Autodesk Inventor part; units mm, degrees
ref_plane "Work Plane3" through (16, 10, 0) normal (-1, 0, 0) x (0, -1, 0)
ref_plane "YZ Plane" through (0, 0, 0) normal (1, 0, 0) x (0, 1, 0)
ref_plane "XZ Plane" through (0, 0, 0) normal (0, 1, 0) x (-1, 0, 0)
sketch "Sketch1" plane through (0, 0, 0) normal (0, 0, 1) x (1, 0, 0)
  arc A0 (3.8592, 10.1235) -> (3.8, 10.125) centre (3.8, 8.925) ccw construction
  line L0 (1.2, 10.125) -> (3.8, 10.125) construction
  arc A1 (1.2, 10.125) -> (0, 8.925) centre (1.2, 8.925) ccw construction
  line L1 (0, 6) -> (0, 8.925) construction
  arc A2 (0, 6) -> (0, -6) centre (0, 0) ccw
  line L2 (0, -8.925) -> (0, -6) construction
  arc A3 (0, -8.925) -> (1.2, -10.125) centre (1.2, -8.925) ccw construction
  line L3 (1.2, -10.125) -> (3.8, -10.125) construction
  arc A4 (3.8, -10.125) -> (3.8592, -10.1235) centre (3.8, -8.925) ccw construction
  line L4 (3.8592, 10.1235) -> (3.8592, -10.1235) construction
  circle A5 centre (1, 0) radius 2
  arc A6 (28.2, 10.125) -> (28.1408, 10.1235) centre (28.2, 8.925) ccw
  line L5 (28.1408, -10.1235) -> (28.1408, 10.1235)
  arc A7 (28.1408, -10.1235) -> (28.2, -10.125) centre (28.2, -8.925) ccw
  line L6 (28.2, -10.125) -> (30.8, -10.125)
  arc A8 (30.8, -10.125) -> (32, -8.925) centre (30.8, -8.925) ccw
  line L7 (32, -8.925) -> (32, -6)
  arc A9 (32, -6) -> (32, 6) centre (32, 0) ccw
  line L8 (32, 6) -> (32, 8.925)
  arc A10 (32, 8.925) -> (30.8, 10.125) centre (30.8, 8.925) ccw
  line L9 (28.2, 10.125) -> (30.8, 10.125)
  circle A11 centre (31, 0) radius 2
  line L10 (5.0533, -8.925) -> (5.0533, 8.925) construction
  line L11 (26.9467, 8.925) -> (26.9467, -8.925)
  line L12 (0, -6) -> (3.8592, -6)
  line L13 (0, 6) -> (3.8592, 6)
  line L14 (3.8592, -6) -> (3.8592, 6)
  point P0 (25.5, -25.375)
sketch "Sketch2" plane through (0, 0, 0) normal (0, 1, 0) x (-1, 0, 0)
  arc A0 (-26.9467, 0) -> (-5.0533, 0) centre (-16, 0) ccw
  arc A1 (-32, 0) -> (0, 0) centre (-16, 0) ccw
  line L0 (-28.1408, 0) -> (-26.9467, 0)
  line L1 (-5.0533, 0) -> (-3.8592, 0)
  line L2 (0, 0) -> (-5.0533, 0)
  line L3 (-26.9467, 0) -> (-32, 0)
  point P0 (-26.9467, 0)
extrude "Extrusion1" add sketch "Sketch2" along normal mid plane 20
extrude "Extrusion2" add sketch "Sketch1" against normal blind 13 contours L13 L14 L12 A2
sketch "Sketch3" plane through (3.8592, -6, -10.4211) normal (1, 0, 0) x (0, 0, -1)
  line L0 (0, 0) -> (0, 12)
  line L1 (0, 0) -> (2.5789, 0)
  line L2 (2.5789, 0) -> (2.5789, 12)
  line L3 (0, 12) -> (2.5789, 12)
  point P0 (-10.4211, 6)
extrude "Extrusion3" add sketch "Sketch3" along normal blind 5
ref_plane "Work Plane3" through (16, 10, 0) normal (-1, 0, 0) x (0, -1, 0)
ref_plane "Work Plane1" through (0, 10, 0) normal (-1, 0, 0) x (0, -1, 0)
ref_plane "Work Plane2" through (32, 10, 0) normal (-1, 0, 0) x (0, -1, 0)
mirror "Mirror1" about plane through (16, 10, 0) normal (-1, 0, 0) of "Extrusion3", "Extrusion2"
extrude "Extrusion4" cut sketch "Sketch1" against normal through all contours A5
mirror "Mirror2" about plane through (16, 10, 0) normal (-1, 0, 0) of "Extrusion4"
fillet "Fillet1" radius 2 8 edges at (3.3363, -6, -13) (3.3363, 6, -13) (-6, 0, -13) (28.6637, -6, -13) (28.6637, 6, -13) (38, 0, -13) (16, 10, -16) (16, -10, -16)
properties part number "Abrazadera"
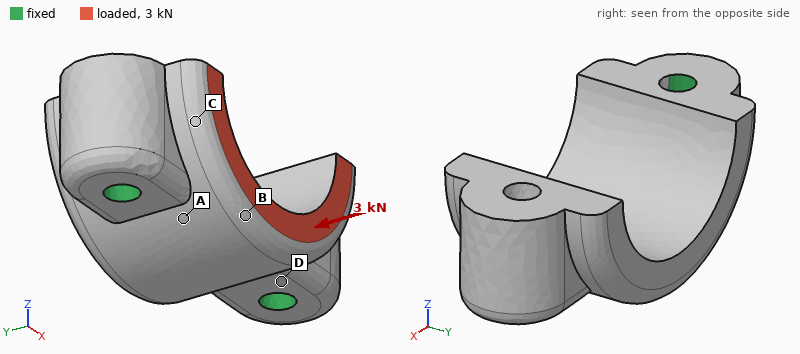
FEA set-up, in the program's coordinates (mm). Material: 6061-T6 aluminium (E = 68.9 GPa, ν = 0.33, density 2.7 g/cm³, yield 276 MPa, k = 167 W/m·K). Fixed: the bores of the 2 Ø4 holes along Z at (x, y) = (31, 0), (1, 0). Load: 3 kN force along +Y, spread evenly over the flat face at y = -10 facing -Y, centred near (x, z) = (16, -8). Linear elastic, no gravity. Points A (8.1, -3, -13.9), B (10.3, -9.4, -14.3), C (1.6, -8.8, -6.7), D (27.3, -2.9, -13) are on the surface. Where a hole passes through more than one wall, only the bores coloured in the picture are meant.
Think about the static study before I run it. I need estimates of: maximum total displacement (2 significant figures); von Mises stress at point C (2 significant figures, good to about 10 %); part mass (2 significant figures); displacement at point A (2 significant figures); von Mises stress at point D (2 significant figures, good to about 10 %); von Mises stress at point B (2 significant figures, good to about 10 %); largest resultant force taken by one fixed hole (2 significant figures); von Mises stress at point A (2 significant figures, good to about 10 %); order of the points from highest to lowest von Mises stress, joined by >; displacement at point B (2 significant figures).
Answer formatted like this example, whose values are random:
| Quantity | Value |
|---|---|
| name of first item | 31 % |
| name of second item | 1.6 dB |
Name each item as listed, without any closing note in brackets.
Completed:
| Quantity | Value |
|---|---|
| maximum total displacement | 12 µm |
| von Mises stress at point C | 7.0 MPa |
| part mass | 16 g |
| displacement at point A | 6.1 µm |
| von Mises stress at point D | 34 MPa |
| von Mises stress at point B | 13 MPa |
| largest resultant force taken by one fixed hole | 1.5 kN |
| von Mises stress at point A | 24 MPa |
| order of the points from highest to lowest von Mises stress, joined by > | D > A > B > C |
| displacement at point B | 7.7 µm |
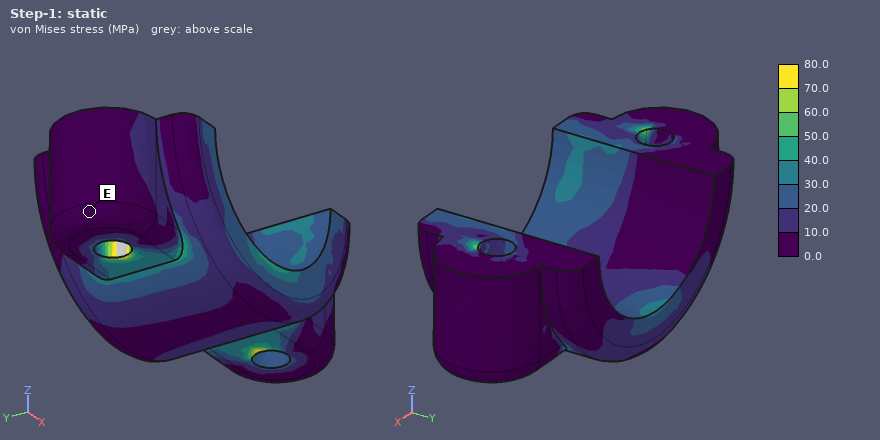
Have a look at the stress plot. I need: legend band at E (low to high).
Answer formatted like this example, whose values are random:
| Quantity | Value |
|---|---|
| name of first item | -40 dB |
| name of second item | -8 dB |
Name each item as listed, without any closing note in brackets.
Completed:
| Quantity | Value |
|---|---|
| legend band at E | 0.0 to 10.0 MPa |
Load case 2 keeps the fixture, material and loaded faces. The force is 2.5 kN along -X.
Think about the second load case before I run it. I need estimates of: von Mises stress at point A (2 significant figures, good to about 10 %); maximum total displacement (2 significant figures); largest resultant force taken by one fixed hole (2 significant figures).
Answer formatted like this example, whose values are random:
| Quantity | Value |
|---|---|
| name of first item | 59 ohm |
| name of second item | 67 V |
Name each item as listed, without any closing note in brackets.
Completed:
| Quantity | Value |
|---|---|
| von Mises stress at point A | 15 MPa |
| maximum total displacement | 15 µm |
| largest resultant force taken by one fixed hole | 1.4 kN |
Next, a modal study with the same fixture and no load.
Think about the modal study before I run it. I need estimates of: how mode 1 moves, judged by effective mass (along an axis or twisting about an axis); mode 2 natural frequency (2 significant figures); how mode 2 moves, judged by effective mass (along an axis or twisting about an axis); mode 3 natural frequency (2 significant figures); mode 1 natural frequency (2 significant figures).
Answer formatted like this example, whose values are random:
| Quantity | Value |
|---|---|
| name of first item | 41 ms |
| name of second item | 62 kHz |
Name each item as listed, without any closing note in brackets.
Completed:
| Quantity | Value |
|---|---|
| how mode 1 moves, judged by effective mass | along Y |
| mode 2 natural frequency | 36 kHz |
| how mode 2 moves, judged by effective mass | along Z |
| mode 3 natural frequency | 41 kHz |
| mode 1 natural frequency | 29 kHz |
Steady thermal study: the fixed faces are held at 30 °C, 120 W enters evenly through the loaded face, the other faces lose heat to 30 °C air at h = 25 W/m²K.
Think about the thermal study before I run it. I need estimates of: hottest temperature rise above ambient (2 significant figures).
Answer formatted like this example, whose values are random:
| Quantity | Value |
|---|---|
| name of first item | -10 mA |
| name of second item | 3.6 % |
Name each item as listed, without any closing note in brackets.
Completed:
| Quantity | Value |
|---|---|
| hottest temperature rise above ambient | 51 K |
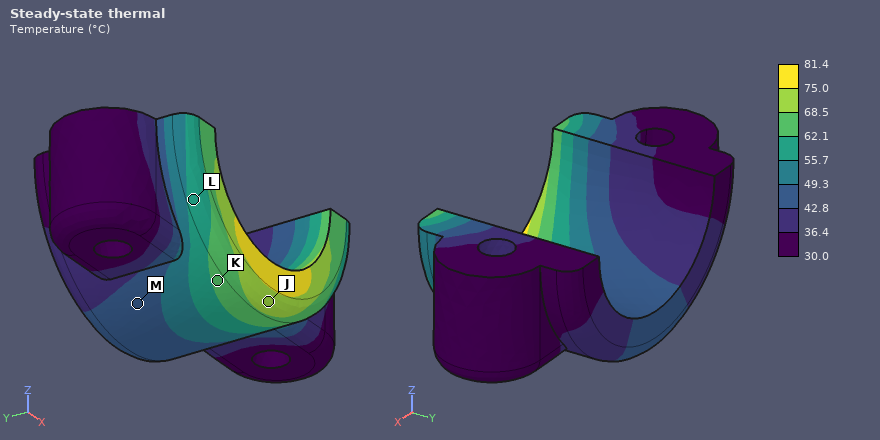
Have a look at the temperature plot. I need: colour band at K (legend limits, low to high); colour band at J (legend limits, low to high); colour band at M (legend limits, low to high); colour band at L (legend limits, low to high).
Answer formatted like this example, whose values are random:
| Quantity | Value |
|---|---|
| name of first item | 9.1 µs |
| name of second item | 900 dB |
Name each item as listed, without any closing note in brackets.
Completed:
| Quantity | Value |
|---|---|
| colour band at K | 62.1 to 68.5 °C |
| colour band at J | 68.5 to 75.0 °C |
| colour band at M | 42.8 to 49.3 °C |
| colour band at L | 55.7 to 62.1 °C |
